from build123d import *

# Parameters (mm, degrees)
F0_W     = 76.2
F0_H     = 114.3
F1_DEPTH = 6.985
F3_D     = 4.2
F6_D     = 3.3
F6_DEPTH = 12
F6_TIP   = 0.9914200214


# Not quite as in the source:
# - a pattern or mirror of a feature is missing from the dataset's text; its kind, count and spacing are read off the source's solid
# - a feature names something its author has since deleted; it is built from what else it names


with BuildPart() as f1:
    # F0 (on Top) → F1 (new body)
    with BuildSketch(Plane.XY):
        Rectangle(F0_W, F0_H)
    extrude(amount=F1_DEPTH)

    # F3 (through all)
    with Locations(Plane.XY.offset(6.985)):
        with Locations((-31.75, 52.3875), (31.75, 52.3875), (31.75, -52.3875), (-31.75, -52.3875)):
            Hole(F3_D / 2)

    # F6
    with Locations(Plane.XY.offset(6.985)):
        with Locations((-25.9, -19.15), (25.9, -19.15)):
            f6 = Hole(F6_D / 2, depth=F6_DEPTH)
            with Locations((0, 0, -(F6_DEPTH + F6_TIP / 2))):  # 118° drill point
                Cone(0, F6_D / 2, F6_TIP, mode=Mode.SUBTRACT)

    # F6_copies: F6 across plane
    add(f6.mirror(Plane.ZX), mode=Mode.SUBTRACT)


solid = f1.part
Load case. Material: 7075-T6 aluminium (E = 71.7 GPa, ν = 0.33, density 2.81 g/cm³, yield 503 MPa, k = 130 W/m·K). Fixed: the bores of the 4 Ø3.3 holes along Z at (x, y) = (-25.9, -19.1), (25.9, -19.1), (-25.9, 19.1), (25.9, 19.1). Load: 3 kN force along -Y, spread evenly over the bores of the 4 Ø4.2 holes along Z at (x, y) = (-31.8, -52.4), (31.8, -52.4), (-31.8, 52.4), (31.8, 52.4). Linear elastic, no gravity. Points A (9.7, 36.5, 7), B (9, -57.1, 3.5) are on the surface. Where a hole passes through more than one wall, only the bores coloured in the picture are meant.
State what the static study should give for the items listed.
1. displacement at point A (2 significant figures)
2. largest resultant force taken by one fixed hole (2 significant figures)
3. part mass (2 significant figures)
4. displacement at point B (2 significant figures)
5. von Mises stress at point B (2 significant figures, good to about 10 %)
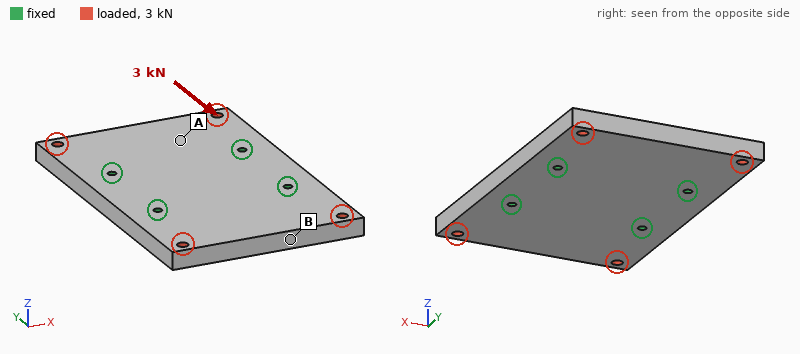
0.83 µm
750 N
170 g
1.0 µm
3.7 MPa
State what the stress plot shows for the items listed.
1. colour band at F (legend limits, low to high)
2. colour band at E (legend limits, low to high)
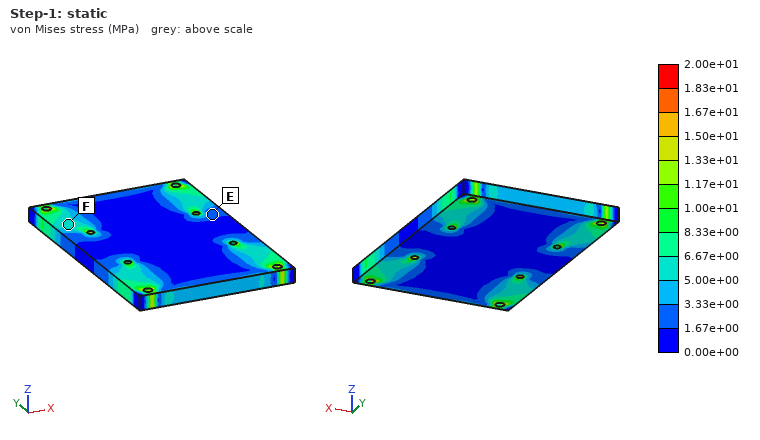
5.00e+00 to 6.67e+00 MPa
1.67e+00 to 3.33e+00 MPa
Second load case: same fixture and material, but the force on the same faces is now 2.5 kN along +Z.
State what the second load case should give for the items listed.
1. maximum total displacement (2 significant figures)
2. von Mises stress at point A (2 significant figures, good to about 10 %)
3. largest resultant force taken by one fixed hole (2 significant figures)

0.18 mm
26 MPa
630 N
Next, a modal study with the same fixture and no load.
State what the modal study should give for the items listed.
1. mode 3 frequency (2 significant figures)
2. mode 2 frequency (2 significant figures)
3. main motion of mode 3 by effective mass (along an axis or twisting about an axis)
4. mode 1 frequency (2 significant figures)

5500 Hz
3300 Hz
twisting about Y
3200 Hz
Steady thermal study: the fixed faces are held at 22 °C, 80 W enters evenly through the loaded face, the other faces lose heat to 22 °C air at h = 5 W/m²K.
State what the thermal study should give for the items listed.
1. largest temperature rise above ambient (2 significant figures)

36 K
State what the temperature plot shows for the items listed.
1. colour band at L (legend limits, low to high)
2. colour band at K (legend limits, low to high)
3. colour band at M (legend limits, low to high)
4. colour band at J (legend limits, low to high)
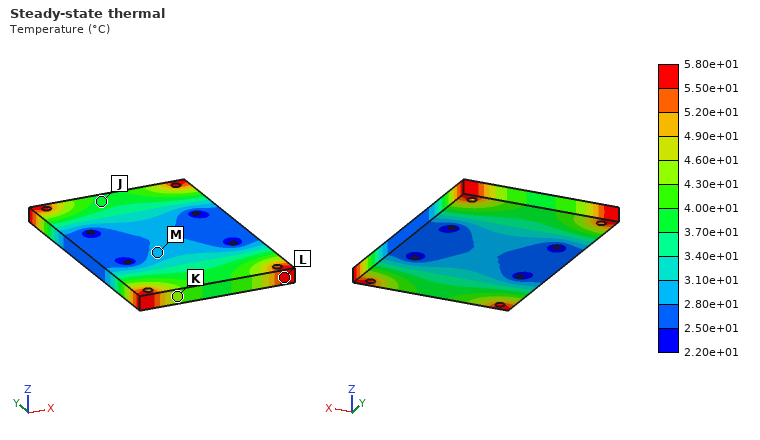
5.50e+01 to 5.80e+01 °C
4.30e+01 to 4.60e+01 °C
2.80e+01 to 3.10e+01 °C
3.70e+01 to 4.00e+01 °C
